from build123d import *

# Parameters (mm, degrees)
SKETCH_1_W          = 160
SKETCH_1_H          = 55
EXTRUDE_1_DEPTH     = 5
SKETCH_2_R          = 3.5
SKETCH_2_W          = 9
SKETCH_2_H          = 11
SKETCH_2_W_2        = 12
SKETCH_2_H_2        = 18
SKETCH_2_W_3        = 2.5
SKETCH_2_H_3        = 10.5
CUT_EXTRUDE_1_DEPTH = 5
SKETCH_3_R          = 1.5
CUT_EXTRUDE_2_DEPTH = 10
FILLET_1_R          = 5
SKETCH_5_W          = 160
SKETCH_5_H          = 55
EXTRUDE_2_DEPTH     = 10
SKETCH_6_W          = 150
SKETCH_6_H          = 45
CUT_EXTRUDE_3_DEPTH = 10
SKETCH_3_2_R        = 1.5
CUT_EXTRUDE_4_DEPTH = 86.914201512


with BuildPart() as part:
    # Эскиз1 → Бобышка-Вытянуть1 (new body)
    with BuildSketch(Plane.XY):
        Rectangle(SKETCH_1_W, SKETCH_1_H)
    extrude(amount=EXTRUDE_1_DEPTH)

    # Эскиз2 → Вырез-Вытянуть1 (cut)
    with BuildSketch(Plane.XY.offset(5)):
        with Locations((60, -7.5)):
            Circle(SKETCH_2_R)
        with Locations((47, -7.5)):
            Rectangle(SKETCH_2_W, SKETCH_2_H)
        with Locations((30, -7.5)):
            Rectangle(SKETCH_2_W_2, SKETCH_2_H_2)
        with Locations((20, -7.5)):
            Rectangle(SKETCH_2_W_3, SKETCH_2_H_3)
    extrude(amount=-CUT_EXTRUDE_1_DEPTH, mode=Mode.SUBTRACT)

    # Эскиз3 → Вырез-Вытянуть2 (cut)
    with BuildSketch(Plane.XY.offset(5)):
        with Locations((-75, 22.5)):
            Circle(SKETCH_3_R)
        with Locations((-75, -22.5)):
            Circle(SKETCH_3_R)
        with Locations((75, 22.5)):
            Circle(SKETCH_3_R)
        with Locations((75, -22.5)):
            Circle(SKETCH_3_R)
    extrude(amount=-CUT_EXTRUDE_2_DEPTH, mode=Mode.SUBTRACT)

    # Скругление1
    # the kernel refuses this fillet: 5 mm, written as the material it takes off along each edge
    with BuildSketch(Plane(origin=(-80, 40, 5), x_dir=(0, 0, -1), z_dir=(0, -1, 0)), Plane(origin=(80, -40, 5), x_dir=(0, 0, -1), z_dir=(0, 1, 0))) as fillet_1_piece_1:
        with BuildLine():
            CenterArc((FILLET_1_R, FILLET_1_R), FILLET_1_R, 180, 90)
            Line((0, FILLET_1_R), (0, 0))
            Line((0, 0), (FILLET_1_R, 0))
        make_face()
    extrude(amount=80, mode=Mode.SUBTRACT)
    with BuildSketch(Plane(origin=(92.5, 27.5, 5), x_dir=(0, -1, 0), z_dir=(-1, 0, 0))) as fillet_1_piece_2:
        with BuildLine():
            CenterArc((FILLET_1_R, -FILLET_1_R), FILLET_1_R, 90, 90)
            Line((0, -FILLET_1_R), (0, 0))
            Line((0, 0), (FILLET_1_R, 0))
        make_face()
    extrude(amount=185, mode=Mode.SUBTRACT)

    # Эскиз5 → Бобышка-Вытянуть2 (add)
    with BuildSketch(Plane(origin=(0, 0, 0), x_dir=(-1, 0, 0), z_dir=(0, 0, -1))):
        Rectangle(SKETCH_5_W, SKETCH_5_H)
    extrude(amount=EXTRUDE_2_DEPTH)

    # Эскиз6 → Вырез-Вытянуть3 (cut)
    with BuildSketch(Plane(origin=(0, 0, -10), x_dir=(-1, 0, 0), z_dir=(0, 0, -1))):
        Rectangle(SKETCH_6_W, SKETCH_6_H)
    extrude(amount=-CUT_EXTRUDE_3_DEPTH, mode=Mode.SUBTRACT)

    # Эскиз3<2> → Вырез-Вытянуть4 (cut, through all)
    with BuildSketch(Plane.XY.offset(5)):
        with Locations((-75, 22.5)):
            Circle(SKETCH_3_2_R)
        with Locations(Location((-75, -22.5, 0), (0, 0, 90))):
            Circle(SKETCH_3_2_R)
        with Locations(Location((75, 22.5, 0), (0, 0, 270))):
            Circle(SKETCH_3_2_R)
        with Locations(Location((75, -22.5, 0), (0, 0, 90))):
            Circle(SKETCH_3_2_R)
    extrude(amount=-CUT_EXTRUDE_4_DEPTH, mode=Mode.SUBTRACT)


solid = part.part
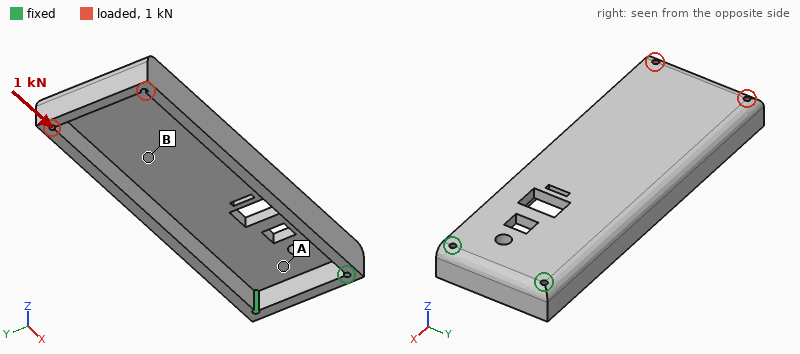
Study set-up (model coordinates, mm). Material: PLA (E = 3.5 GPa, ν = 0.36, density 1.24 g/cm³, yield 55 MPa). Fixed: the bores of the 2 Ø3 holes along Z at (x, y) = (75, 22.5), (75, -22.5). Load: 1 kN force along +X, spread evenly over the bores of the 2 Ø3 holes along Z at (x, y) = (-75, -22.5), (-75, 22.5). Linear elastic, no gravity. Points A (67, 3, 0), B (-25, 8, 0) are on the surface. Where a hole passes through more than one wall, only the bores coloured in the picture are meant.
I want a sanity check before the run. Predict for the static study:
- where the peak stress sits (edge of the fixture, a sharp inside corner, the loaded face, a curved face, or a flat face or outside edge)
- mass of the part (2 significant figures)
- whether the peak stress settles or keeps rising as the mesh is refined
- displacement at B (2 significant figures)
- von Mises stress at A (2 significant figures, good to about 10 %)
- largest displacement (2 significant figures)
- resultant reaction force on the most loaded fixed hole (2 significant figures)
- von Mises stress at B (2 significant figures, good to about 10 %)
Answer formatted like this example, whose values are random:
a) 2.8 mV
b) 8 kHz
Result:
a) edge of the fixture
b) 75 g
c) keeps rising
d) 0.57 mm
e) 1.4 MPa
f) 1.4 mm
g) 500 N
h) 2.8 MPa
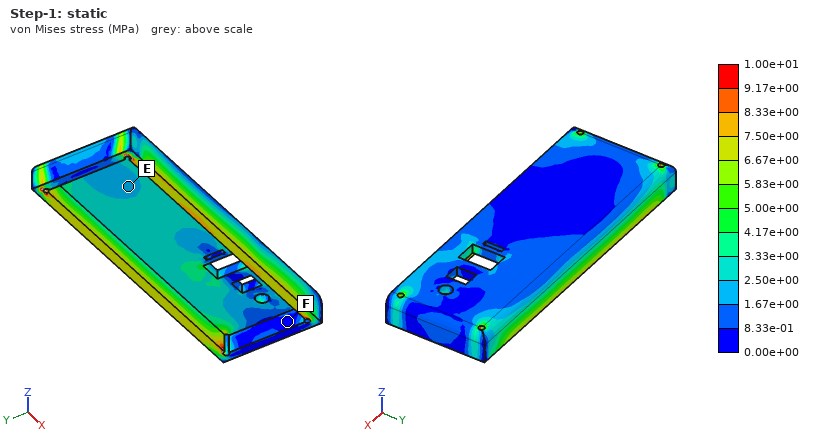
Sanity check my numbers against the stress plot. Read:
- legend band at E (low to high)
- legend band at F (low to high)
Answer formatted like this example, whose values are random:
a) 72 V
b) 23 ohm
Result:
a) 1.67e+00 to 2.50e+00 MPa
b) 0.00e+00 to 8.33e-01 MPa
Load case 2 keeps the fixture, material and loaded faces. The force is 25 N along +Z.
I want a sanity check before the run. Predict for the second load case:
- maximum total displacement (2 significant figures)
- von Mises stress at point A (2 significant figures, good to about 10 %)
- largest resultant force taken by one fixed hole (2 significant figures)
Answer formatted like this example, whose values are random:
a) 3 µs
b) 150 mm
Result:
a) 1.8 mm
b) 1.4 MPa
c) 39 N
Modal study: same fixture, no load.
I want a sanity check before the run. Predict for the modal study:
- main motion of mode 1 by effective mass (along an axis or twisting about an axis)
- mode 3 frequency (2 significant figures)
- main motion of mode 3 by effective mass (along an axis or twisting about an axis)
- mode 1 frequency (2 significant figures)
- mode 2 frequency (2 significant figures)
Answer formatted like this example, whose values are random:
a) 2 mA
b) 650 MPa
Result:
a) along Z
b) 590 Hz
c) along Y
d) 130 Hz
e) 310 Hz
